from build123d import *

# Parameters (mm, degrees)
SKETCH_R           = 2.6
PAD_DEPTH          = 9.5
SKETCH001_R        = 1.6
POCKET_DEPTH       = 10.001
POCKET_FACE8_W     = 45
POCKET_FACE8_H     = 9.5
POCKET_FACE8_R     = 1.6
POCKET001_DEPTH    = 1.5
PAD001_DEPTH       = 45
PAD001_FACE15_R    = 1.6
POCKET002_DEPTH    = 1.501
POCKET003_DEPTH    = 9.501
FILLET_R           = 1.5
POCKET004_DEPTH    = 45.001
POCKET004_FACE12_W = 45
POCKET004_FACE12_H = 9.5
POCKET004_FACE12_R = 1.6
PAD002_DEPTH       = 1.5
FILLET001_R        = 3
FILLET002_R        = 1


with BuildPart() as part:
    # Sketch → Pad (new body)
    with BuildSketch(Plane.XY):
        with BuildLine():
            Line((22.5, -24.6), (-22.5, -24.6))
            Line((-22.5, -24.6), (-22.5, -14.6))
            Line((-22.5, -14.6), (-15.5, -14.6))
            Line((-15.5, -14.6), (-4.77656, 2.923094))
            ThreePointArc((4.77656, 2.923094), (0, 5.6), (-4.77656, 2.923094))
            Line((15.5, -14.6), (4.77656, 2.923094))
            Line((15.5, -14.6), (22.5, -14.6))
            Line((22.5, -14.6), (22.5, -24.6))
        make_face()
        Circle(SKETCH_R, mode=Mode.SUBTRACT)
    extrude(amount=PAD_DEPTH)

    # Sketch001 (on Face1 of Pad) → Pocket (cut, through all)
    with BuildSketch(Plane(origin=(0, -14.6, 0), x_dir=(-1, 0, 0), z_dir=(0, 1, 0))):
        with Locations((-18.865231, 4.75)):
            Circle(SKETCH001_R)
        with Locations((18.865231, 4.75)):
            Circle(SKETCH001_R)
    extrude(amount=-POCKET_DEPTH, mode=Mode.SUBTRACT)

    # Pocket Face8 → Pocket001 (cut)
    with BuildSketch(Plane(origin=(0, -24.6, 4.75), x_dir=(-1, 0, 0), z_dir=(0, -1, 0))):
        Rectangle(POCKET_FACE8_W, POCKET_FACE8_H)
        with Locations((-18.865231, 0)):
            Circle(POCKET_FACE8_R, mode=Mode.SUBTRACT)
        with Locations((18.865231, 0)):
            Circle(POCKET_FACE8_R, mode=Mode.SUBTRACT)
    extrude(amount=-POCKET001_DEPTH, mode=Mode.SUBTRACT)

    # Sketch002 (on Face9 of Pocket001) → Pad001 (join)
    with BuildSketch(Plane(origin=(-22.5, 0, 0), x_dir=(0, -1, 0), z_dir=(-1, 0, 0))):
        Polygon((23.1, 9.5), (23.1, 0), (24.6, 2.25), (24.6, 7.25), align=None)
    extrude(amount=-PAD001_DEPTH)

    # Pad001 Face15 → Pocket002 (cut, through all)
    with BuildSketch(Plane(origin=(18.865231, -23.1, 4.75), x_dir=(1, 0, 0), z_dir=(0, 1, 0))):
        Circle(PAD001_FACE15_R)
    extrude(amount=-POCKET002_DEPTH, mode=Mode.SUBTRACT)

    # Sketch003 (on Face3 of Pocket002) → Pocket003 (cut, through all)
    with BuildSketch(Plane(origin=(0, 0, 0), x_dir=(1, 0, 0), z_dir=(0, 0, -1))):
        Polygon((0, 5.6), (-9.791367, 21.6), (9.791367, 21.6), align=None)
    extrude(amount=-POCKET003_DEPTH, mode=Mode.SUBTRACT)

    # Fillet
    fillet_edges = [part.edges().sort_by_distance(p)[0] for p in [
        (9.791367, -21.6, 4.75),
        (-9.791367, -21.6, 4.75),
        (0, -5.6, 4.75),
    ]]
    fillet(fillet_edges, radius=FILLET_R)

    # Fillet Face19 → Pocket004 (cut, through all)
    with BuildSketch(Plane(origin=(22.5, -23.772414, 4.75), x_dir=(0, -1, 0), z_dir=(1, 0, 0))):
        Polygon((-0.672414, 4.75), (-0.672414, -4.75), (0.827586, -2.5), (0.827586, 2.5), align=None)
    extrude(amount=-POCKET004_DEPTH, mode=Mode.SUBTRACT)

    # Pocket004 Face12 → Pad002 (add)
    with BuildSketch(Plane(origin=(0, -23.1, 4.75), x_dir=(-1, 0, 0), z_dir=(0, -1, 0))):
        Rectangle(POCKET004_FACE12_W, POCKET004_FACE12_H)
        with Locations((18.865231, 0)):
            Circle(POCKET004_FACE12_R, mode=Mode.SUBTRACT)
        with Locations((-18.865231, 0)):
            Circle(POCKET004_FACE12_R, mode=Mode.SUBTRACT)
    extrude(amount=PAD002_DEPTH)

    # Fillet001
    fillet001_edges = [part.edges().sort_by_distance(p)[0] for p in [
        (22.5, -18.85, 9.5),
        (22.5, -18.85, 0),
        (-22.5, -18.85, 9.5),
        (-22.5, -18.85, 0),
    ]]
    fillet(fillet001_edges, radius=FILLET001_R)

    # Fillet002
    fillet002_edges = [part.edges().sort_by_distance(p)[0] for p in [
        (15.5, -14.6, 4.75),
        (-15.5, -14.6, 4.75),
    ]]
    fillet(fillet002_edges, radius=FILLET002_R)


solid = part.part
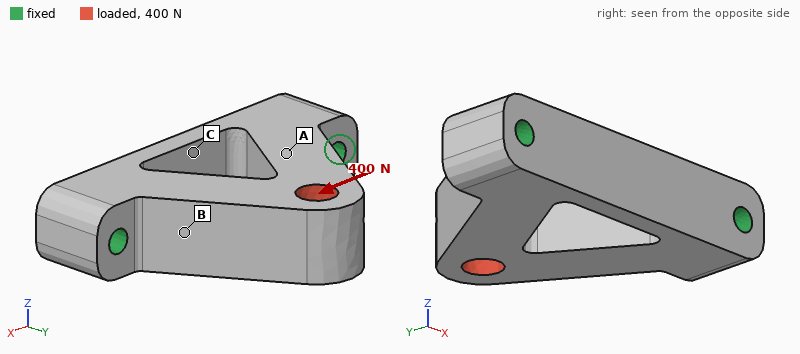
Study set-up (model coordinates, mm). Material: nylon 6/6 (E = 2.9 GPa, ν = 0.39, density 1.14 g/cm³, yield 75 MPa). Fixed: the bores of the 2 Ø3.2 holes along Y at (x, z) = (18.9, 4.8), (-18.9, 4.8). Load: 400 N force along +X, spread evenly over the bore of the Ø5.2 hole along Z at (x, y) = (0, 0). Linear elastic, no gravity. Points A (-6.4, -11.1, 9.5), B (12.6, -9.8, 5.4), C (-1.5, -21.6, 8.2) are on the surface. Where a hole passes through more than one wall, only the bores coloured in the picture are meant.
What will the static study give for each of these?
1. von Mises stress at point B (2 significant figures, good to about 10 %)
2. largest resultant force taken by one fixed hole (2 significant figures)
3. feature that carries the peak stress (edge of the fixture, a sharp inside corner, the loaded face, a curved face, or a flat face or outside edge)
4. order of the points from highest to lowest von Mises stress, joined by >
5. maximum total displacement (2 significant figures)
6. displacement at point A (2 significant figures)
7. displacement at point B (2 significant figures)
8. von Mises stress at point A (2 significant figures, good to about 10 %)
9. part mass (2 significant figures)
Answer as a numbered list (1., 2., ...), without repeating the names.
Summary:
1. 6.9 MPa
2. 300 N
3. a curved face
4. B > A > C
5. 92 µm
6. 22 µm
7. 30 µm
8. 3.3 MPa
9. 6.8 g
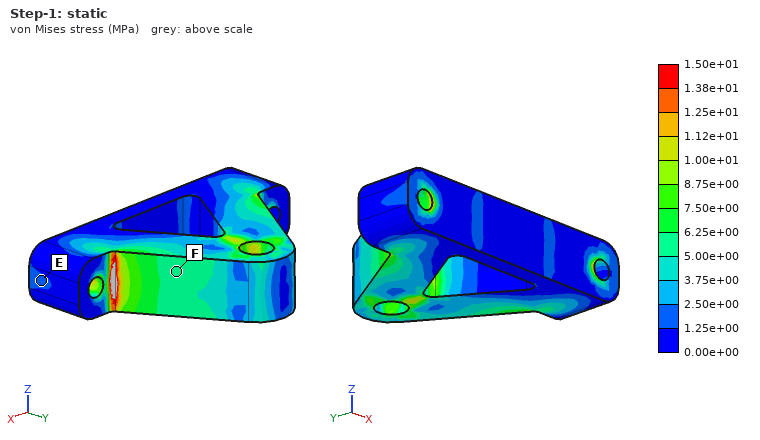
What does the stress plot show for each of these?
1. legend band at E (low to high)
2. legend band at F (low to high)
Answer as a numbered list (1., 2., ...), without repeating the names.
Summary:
1. 1.25e+00 to 2.50e+00 MPa
2. 5.00e+00 to 6.25e+00 MPa
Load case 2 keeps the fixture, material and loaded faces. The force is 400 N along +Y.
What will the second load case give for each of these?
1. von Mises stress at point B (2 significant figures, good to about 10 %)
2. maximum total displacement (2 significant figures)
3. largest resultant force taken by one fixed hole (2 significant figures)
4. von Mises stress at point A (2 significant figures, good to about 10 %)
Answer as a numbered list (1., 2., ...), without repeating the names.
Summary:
1. 3.9 MPa
2. 46 µm
3. 230 N
4. 2.8 MPa
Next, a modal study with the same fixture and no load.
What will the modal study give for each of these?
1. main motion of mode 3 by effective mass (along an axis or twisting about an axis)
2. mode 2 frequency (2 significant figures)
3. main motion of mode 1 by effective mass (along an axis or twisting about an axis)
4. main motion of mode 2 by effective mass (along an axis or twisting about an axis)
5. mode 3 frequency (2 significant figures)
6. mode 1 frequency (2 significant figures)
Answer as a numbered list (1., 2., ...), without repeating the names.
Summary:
1. along Y
2. 8000 Hz
3. along Z
4. along Z
5. 8400 Hz
6. 2900 Hz
